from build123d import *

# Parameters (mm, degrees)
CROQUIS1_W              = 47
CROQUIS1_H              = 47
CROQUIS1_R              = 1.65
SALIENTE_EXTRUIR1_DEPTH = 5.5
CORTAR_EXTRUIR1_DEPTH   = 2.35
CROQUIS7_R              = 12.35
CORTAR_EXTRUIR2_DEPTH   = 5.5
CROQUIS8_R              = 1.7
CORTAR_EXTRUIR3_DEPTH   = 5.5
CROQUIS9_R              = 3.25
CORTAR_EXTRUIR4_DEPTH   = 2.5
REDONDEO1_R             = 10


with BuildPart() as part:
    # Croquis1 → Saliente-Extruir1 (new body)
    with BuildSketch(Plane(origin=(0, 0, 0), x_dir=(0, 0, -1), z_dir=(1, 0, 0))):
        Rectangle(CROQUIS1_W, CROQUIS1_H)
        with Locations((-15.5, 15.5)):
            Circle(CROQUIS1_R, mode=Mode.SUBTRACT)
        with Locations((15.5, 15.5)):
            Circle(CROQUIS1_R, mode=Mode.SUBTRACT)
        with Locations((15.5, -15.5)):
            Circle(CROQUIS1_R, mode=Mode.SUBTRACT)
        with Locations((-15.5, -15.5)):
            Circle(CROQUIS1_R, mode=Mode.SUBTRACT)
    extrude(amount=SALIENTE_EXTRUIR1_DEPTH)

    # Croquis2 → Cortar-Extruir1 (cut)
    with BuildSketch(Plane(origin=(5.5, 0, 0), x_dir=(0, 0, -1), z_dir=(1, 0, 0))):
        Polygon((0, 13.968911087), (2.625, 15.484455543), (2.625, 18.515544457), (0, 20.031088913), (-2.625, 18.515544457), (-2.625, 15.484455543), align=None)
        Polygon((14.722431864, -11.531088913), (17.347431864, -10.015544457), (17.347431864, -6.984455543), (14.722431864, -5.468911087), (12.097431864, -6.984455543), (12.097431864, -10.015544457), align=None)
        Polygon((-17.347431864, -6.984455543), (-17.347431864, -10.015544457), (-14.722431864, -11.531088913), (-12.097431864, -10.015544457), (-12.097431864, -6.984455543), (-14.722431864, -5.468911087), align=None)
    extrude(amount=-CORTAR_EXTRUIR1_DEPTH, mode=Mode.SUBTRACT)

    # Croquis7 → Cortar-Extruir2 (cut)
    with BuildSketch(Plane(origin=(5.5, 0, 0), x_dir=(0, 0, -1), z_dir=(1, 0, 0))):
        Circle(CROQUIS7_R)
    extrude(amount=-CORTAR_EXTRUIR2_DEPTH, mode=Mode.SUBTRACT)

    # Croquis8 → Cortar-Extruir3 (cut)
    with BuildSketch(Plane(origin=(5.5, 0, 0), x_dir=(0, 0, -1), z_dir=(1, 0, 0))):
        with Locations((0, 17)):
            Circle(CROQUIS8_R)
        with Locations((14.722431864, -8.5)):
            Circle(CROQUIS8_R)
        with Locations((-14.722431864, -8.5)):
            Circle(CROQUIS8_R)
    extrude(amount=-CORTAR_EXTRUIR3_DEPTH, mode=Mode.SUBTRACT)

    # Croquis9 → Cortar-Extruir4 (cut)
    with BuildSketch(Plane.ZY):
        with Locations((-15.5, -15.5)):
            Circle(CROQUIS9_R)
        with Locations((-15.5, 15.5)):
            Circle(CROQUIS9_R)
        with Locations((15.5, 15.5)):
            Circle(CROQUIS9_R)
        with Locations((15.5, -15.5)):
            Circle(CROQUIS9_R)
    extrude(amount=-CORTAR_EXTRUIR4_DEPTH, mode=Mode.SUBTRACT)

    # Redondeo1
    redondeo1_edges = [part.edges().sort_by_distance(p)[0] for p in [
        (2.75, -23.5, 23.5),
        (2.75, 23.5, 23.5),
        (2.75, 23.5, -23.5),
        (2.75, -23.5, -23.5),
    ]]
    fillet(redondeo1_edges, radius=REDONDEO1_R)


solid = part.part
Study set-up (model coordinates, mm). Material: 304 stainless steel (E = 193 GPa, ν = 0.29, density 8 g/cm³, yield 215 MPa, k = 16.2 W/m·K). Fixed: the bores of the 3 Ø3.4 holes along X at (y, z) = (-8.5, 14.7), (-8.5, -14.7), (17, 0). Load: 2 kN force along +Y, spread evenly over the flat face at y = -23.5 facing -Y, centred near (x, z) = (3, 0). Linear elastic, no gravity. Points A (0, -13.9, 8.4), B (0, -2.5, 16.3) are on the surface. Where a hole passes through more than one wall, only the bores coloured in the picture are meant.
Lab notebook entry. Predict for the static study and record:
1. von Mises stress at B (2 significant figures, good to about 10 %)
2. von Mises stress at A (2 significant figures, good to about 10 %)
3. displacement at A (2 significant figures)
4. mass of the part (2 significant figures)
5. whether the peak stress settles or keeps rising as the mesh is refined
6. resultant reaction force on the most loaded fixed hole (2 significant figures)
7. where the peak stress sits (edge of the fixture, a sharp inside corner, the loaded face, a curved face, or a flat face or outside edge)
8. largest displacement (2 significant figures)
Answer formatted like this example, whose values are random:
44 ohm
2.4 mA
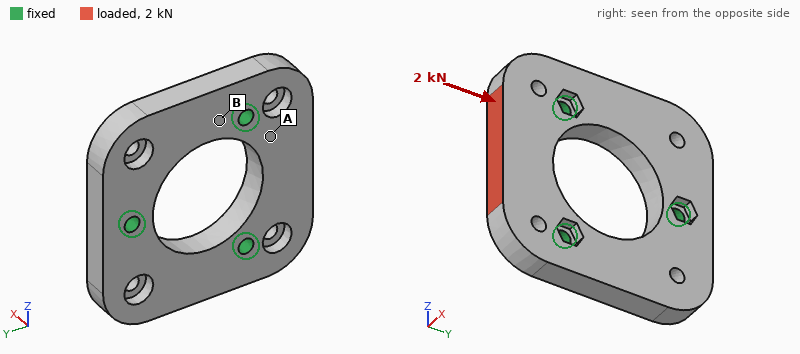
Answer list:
9.7 MPa
27 MPa
2.0 µm
67 g
keeps rising
1.1 kN
edge of the fixture
4.9 µm
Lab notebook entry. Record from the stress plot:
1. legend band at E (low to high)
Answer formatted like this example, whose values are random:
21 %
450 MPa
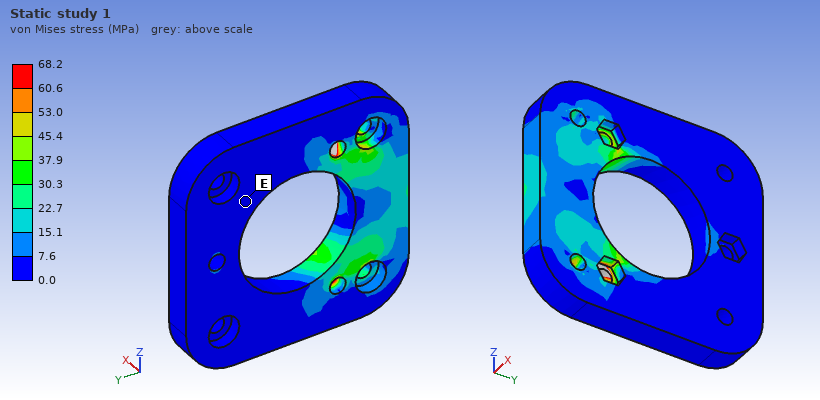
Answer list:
0.0 to 7.6 MPa
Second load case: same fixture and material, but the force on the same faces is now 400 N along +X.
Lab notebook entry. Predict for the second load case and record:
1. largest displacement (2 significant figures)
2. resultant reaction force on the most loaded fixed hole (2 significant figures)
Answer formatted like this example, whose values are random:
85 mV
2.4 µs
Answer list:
17 µm
230 N
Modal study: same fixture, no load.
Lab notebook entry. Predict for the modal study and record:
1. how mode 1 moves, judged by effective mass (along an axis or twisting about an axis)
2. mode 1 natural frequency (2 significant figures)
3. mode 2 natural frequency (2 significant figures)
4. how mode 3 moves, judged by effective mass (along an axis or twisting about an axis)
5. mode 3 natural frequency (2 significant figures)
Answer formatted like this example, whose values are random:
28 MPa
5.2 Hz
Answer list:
twisting about Y
7900 Hz
8500 Hz
along X
11 kHz
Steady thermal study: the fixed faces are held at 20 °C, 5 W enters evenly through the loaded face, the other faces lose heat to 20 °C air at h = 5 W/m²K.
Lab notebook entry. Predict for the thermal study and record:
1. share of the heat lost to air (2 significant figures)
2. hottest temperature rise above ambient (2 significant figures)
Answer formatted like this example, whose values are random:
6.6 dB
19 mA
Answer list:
4.1 %
42 K
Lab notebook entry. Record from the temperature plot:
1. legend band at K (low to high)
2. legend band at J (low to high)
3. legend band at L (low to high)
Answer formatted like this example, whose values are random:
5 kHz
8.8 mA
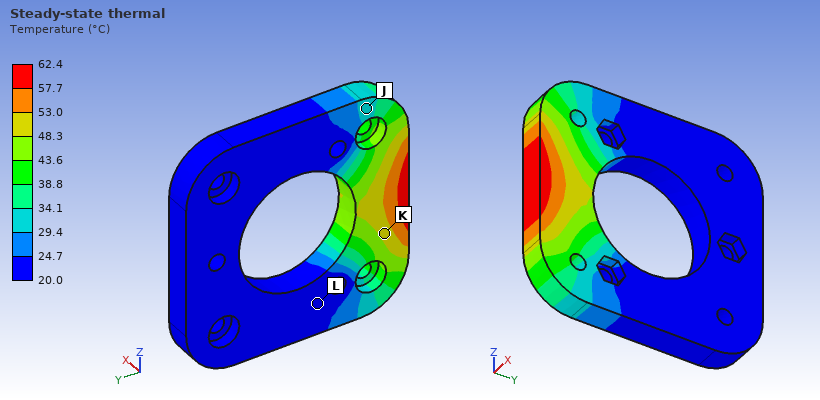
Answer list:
48.3 to 53.0 °C
29.4 to 34.1 °C
20.0 to 24.7 °C
